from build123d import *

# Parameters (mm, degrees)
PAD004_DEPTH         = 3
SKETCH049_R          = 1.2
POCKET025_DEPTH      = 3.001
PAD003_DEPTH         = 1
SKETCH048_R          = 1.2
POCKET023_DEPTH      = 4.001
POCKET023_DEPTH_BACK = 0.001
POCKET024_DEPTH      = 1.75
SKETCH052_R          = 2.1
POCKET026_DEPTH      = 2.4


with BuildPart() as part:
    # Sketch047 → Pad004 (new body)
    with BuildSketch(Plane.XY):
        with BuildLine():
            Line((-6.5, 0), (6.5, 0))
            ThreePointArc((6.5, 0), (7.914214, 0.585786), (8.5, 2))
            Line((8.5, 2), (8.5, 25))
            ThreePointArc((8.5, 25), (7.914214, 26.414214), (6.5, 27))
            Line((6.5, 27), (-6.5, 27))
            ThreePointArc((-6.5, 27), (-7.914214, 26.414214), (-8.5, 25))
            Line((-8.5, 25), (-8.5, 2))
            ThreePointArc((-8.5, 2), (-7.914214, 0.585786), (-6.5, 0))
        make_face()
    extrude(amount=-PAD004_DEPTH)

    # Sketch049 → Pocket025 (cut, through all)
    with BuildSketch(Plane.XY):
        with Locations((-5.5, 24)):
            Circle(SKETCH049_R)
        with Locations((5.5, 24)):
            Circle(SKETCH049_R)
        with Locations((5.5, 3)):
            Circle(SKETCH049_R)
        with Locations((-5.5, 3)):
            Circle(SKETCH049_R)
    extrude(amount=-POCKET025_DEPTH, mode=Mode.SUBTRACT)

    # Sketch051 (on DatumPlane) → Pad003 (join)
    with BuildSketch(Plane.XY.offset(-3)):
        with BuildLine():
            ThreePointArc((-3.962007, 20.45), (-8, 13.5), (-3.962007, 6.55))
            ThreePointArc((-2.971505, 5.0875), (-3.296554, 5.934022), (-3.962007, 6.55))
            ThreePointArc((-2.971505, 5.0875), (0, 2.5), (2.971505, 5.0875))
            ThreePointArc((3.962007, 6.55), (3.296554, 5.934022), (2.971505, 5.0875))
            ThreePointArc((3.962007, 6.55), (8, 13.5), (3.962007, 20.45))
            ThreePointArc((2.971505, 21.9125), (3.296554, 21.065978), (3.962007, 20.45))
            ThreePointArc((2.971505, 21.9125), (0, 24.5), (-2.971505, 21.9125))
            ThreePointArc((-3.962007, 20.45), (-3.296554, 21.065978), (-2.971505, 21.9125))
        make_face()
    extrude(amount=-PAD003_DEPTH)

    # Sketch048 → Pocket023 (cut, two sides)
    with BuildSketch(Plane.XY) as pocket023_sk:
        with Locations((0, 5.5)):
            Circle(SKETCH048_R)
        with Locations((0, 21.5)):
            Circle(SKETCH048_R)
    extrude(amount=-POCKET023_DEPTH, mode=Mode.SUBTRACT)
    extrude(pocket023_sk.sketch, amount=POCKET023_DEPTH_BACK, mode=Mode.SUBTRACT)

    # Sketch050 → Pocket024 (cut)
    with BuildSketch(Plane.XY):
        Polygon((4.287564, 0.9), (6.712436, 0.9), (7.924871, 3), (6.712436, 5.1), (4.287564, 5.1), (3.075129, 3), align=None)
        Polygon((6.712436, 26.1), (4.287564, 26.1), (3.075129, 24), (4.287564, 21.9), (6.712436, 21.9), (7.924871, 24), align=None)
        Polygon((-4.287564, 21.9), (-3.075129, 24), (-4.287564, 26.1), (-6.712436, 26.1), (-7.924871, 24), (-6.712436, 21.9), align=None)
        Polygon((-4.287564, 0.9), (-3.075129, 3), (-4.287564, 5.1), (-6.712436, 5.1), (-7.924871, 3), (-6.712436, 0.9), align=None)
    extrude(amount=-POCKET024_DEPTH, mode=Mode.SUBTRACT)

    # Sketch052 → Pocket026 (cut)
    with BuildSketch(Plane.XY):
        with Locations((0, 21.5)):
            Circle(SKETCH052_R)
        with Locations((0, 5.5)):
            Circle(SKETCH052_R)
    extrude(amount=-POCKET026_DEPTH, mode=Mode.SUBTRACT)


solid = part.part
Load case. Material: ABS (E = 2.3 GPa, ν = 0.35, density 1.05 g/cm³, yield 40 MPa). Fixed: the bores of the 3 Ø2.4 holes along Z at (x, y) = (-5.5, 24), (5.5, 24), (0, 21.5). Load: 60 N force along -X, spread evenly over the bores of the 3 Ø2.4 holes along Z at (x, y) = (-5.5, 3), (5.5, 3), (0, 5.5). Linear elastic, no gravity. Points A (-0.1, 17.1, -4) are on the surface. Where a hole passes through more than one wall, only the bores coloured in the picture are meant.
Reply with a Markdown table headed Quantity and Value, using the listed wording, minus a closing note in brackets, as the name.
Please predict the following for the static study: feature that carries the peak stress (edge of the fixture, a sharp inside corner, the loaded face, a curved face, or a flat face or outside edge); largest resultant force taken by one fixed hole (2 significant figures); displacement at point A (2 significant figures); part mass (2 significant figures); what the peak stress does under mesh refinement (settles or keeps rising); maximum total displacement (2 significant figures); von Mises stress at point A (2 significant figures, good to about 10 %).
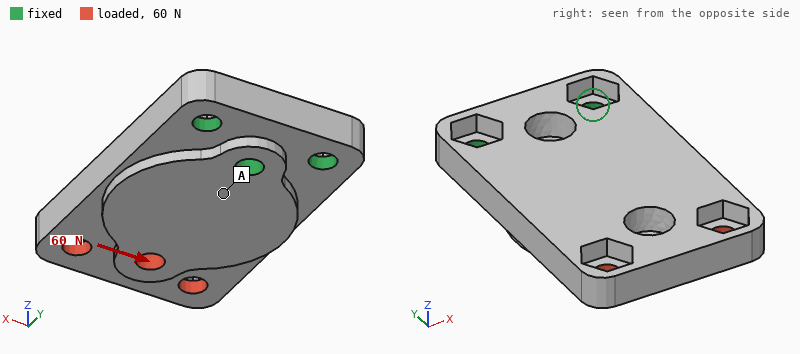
| Quantity | Value |
|---|---|
| feature that carries the peak stress | edge of the fixture |
| largest resultant force taken by one fixed hole | 82 N |
| displacement at point A | 0.025 mm |
| part mass | 1.5 g |
| what the peak stress does under mesh refinement | keeps rising |
| maximum total displacement | 0.14 mm |
| von Mises stress at point A | 3.7 MPa |
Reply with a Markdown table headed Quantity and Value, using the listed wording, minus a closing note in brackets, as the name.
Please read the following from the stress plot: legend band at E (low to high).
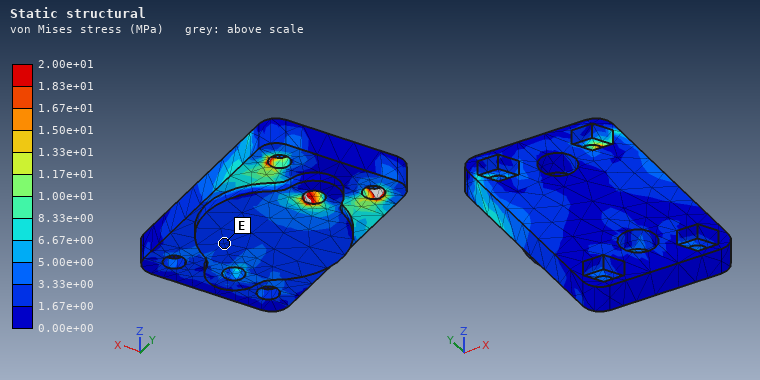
| Quantity | Value |
|---|---|
| legend band at E | 1.67e+00 to 3.33e+00 MPa |
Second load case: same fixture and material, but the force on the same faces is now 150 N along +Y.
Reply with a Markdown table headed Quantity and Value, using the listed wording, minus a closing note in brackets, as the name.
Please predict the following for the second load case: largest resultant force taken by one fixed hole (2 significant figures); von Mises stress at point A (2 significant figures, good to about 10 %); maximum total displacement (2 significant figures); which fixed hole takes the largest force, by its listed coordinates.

| Quantity | Value |
|---|---|
| largest resultant force taken by one fixed hole | 74 N |
| von Mises stress at point A | 7.0 MPa |
| maximum total displacement | 0.14 mm |
| which fixed hole takes the largest force, by its listed coordinates | (0, 21.5) |
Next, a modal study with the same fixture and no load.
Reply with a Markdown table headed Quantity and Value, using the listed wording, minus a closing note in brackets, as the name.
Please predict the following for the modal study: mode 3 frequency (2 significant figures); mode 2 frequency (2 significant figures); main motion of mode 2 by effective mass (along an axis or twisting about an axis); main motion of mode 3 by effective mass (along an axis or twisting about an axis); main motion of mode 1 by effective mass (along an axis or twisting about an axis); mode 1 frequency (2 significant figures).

| Quantity | Value |
|---|---|
| mode 3 frequency | 5100 Hz |
| mode 2 frequency | 4400 Hz |
| main motion of mode 2 by effective mass | twisting about Y |
| main motion of mode 3 by effective mass | along X |
| main motion of mode 1 by effective mass | along Z |
| mode 1 frequency | 1700 Hz |
